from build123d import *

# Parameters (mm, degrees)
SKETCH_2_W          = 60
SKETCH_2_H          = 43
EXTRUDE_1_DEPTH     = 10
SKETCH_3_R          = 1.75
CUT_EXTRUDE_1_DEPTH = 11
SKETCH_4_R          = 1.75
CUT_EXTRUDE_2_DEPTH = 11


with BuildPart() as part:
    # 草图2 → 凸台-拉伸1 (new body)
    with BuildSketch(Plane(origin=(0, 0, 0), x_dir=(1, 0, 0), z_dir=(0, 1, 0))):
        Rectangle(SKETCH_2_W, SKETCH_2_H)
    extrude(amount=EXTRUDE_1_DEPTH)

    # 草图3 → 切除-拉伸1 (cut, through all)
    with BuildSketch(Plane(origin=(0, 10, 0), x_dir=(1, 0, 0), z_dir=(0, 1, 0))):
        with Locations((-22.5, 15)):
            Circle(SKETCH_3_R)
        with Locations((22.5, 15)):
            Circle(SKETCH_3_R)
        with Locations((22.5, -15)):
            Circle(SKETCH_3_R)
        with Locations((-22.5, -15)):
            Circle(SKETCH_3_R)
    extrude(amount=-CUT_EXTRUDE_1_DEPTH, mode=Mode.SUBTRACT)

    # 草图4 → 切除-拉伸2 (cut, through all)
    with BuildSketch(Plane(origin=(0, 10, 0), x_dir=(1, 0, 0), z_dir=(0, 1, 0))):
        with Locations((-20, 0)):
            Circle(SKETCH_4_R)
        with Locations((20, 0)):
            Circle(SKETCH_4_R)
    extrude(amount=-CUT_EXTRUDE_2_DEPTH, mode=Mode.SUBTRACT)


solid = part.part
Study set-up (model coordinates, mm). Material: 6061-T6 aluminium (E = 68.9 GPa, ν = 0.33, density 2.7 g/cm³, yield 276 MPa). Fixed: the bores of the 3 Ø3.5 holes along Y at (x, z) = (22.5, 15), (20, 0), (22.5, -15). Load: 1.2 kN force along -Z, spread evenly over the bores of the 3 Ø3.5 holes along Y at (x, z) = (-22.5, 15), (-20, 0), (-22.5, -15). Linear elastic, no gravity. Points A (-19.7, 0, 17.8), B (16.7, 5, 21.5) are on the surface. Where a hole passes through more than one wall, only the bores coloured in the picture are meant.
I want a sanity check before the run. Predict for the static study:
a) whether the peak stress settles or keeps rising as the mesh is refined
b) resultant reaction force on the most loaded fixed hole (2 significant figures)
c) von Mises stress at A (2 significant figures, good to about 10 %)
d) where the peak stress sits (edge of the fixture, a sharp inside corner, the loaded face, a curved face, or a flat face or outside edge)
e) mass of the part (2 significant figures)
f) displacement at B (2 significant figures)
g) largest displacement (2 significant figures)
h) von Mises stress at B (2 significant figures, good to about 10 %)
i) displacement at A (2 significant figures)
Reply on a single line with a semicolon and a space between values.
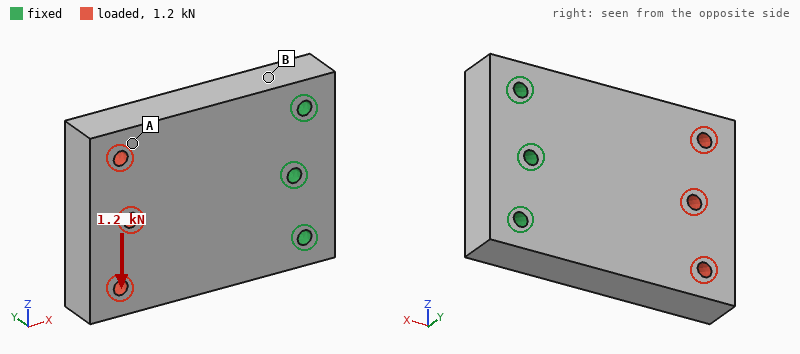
keeps rising; 1.6 kN; 3.7 MPa; edge of the fixture; 68 g; 2.8 µm; 18 µm; 11 MPa; 14 µm
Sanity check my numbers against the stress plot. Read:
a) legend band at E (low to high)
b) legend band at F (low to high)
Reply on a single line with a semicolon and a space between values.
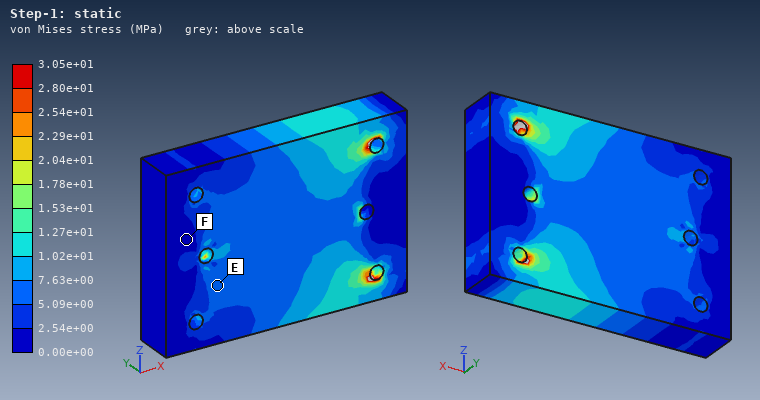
5.09e+00 to 7.63e+00 MPa; 0.00e+00 to 2.54e+00 MPa
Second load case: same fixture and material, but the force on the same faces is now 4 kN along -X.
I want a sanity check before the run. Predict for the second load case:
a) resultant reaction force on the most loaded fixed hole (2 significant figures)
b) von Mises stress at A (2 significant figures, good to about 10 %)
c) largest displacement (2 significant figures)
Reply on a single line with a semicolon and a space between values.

1.4 kN; 12 MPa; 7.0 µm
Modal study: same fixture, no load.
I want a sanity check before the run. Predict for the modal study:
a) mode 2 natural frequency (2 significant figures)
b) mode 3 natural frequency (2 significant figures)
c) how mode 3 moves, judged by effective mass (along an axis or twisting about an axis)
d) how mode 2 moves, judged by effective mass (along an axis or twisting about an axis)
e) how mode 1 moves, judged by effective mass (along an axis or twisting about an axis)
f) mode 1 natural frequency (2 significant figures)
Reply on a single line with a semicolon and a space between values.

7400 Hz; 8800 Hz; along Z; twisting about X; along Y; 3000 Hz
